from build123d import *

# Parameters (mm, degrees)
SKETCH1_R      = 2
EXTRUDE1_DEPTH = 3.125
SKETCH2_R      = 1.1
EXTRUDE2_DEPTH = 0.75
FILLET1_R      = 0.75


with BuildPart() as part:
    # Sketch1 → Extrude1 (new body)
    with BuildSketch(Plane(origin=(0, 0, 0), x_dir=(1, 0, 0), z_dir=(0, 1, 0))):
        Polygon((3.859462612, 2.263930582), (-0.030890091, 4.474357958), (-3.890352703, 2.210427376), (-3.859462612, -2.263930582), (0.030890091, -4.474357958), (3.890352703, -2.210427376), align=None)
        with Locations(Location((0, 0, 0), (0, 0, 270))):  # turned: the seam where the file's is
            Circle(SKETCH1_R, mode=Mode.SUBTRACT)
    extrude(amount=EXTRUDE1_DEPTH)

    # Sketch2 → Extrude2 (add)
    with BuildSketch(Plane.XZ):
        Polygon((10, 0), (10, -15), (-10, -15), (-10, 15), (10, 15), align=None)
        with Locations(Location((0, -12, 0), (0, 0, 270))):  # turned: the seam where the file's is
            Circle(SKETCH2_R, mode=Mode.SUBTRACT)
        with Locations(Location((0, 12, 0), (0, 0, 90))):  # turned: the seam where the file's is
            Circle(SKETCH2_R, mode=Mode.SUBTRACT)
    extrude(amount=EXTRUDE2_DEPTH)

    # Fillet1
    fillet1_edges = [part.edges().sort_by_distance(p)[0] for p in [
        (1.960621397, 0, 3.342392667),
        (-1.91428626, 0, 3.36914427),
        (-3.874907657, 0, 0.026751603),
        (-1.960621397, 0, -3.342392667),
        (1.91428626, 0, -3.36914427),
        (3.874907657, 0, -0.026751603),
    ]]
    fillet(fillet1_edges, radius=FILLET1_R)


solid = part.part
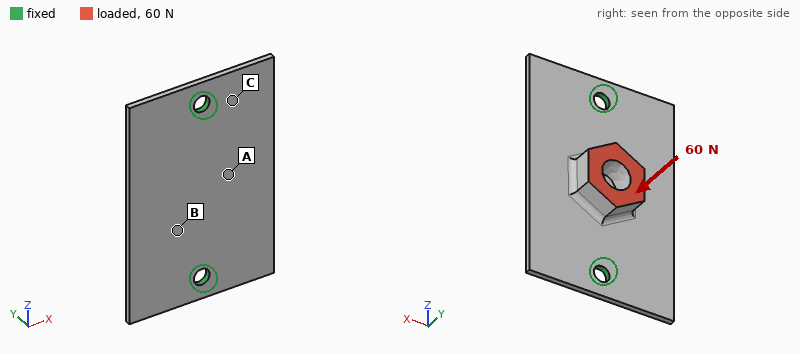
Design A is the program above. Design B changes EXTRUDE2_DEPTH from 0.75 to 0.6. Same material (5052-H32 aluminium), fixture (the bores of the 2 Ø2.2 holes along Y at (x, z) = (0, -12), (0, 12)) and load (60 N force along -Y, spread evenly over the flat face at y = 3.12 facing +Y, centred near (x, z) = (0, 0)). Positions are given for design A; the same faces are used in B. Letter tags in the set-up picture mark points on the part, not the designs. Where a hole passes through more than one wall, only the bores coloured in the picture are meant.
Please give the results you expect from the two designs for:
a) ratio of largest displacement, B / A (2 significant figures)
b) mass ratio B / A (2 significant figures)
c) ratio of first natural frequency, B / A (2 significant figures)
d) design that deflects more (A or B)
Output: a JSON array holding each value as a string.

["1.8", "0.84", "0.80", "B"]
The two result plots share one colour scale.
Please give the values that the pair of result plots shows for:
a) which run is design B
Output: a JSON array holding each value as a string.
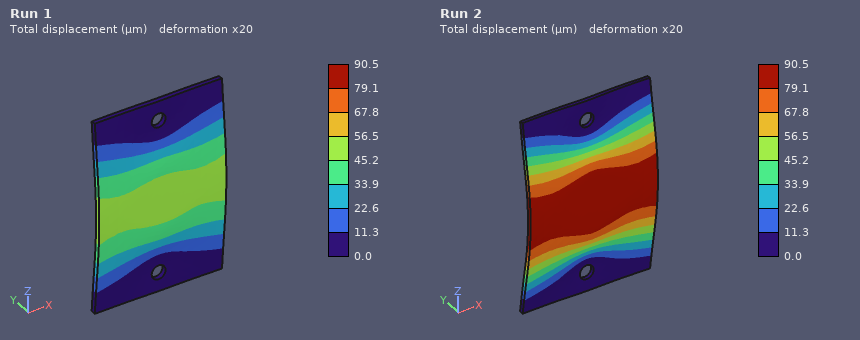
["Run 2"]
